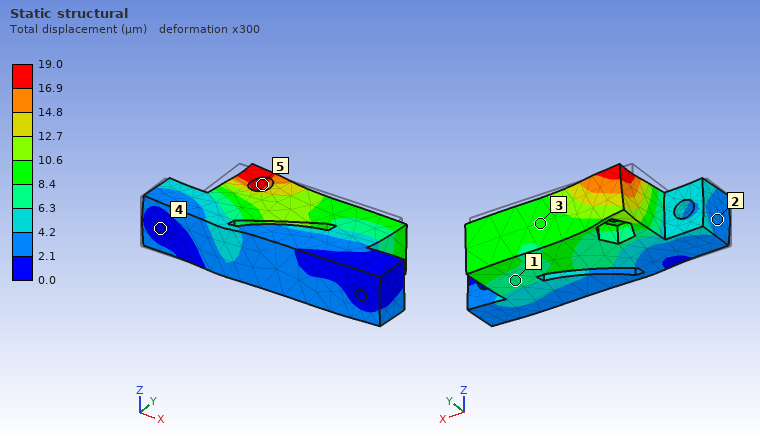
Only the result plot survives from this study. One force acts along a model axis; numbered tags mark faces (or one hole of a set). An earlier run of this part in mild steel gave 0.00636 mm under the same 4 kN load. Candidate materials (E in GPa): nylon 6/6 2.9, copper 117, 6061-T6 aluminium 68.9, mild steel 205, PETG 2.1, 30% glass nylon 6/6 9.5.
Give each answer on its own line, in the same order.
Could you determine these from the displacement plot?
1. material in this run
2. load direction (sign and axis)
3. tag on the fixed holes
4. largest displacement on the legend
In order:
6061-T6 aluminium
+X
4
19.0 µm
